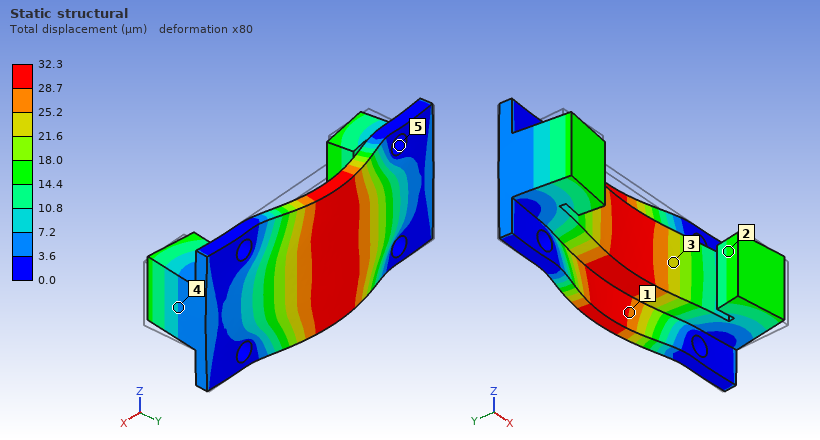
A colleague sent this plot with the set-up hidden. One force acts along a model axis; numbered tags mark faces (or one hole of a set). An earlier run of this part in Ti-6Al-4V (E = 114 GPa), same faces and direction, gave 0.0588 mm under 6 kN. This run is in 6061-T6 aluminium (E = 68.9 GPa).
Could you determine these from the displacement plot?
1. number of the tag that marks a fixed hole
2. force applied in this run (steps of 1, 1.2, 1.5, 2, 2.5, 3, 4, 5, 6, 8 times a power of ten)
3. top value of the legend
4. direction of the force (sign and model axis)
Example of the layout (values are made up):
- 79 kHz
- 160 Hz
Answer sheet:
- 5
- 2 kN
- 32.3 µm
- +Y
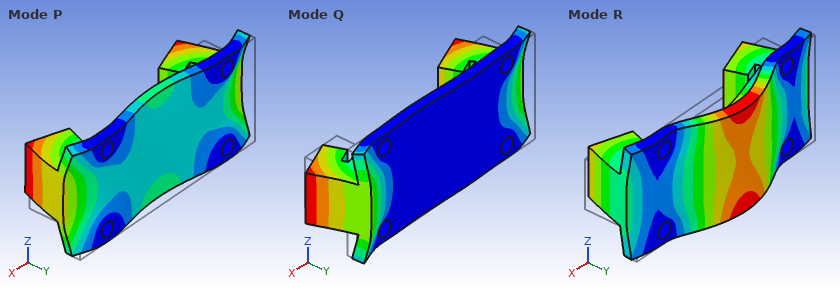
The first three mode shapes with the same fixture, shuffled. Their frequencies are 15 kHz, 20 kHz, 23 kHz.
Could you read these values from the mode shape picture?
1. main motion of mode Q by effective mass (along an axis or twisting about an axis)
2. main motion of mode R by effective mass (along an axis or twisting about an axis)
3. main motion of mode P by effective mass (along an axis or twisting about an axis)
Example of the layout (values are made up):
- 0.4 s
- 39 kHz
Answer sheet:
- along X
- along Y
- along Y
